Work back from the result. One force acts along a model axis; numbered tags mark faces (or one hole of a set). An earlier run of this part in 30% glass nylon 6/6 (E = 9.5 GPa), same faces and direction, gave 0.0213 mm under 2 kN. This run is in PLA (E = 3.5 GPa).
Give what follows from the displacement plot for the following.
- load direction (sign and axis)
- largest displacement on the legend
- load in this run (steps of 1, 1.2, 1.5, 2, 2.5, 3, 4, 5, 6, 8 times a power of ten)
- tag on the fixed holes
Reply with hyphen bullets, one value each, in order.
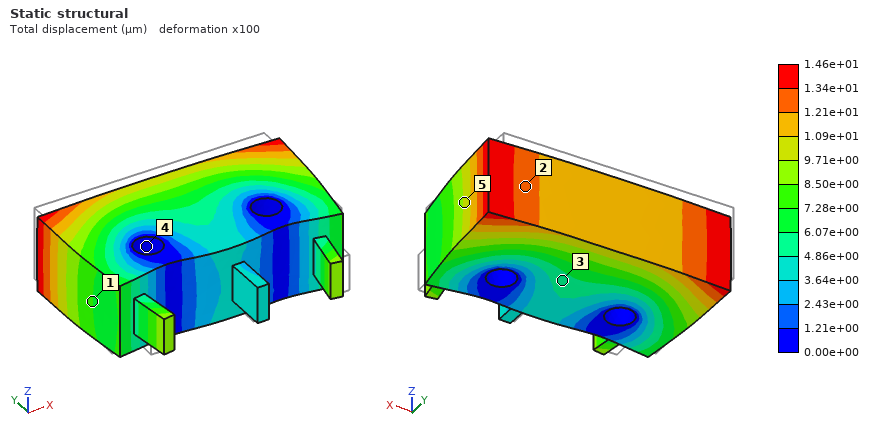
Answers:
- -Y
- 1.46e+01 µm
- 500 N
- 4
